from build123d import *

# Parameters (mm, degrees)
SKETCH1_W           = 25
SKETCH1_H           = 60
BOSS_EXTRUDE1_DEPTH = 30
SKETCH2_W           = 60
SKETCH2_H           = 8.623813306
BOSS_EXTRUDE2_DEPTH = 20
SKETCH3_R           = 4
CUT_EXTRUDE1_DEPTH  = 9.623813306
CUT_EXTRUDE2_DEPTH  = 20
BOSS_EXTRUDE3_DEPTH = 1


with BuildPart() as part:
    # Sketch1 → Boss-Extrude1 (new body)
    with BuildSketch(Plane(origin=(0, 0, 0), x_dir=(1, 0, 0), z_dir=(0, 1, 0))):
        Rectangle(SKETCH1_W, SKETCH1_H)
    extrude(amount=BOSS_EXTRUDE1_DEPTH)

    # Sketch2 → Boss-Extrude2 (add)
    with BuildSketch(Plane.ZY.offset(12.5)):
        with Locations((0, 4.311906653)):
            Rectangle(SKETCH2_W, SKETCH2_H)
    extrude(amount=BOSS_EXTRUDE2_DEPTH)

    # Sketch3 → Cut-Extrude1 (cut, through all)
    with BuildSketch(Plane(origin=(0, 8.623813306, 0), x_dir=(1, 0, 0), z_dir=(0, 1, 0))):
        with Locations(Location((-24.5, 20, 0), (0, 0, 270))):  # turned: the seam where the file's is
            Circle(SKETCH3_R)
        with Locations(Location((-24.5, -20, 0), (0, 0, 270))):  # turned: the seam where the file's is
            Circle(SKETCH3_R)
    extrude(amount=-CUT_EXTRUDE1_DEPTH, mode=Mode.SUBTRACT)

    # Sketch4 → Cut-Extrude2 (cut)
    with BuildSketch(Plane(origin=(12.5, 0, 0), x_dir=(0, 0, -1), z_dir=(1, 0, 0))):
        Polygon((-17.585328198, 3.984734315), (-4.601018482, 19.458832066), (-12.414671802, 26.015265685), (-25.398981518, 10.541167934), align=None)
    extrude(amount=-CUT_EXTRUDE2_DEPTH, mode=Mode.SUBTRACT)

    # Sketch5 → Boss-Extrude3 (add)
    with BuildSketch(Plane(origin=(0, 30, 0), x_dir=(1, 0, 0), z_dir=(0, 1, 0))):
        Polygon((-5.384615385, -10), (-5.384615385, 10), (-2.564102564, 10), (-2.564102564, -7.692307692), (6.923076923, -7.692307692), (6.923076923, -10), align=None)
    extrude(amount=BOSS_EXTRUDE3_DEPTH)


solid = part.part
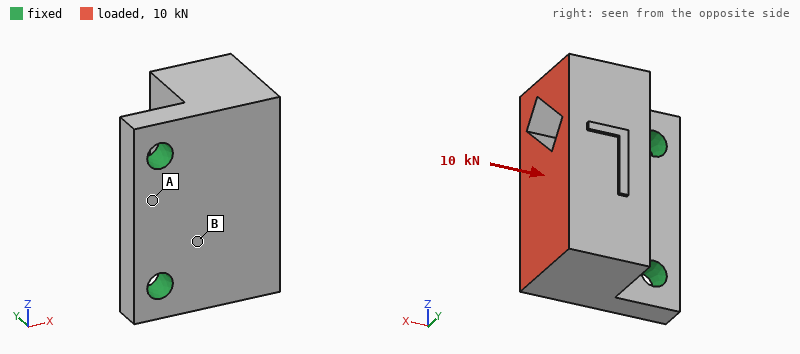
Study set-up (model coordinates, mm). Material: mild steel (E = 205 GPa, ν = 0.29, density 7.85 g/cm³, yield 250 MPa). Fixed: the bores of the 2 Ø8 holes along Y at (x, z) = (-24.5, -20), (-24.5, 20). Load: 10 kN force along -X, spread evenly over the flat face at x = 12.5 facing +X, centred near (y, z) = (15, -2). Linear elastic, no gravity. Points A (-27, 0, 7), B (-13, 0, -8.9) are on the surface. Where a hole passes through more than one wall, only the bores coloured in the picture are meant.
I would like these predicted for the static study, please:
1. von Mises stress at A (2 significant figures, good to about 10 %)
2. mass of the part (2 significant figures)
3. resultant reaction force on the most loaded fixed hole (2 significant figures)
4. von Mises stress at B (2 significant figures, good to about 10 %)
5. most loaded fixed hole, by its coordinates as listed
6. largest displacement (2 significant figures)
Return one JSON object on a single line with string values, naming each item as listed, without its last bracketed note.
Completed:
{"von Mises stress at A": "31 MPa", "mass of the part": "400 g", "resultant reaction force on the most loaded fixed hole": "5.5 kN", "von Mises stress at B": "93 MPa", "most loaded fixed hole, by its coordinates as listed": "(-24.5, -20)", "largest displacement": "0.10 mm"}
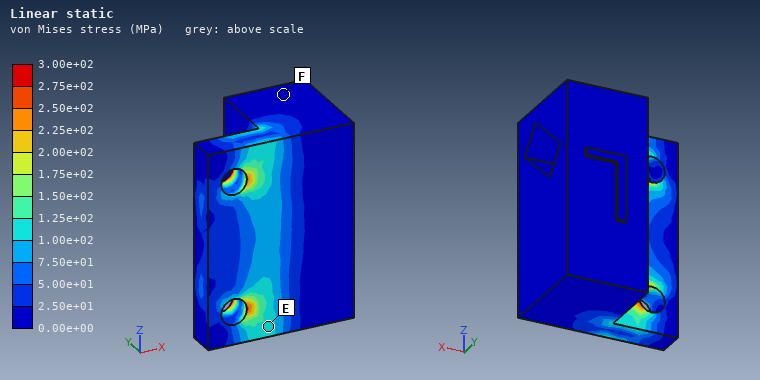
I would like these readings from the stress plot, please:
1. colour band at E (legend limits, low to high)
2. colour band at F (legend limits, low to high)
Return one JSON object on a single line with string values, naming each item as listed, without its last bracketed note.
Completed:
{"colour band at E": "1.00e+02 to 1.25e+02 MPa", "colour band at F": "0.00e+00 to 2.50e+01 MPa"}
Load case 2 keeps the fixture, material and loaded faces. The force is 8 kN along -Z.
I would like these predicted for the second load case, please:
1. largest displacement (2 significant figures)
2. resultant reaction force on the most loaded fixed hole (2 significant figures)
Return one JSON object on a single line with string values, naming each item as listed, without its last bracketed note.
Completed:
{"largest displacement": "18 µm", "resultant reaction force on the most loaded fixed hole": "7.9 kN"}
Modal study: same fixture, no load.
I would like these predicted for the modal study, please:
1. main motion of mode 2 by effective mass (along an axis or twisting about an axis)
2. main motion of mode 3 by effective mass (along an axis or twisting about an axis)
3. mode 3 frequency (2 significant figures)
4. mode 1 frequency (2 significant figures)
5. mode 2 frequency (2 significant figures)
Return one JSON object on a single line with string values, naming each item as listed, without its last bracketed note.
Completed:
{"main motion of mode 2 by effective mass": "along Z", "main motion of mode 3 by effective mass": "along Z", "mode 3 frequency": "10 kHz", "mode 1 frequency": "2500 Hz", "mode 2 frequency": "6900 Hz"}
